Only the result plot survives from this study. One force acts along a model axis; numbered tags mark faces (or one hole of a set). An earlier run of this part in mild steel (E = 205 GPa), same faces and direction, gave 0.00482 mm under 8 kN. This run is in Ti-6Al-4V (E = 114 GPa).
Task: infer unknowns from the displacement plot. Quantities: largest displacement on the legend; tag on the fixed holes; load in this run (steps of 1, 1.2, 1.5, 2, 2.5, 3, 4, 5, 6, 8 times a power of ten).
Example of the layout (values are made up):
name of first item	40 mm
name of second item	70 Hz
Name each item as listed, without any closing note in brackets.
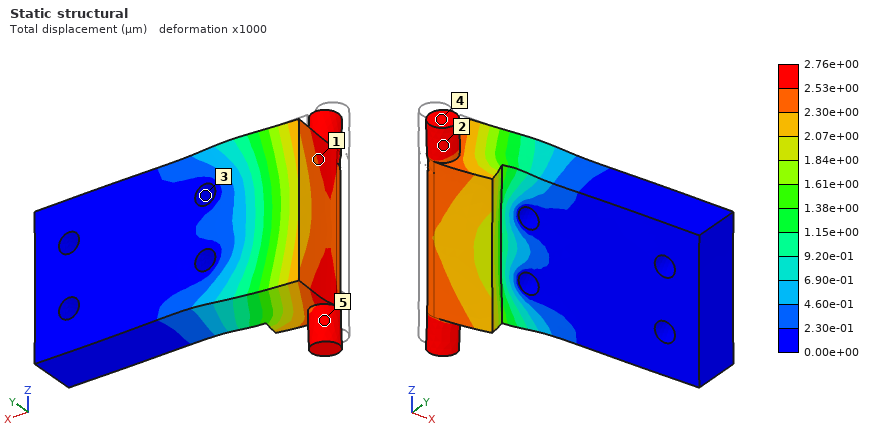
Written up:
largest displacement on the legend	2.76e+00 µm
tag on the fixed holes	3
load in this run	2.5 kN
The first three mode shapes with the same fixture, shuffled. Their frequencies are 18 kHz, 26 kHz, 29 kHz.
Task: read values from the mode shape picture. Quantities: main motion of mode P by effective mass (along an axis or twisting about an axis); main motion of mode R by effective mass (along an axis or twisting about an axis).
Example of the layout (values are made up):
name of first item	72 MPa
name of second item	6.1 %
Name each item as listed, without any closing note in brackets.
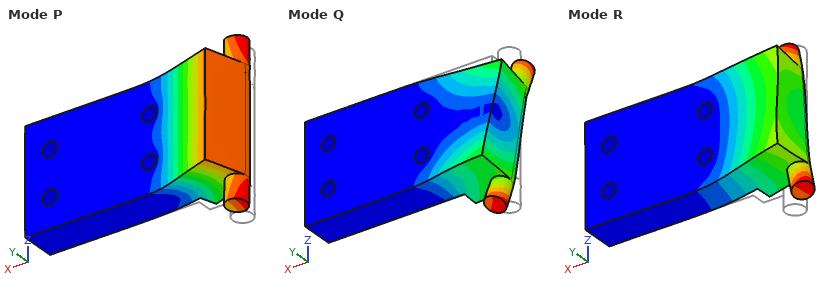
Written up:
main motion of mode P by effective mass	along Y
main motion of mode R by effective mass	along Z
